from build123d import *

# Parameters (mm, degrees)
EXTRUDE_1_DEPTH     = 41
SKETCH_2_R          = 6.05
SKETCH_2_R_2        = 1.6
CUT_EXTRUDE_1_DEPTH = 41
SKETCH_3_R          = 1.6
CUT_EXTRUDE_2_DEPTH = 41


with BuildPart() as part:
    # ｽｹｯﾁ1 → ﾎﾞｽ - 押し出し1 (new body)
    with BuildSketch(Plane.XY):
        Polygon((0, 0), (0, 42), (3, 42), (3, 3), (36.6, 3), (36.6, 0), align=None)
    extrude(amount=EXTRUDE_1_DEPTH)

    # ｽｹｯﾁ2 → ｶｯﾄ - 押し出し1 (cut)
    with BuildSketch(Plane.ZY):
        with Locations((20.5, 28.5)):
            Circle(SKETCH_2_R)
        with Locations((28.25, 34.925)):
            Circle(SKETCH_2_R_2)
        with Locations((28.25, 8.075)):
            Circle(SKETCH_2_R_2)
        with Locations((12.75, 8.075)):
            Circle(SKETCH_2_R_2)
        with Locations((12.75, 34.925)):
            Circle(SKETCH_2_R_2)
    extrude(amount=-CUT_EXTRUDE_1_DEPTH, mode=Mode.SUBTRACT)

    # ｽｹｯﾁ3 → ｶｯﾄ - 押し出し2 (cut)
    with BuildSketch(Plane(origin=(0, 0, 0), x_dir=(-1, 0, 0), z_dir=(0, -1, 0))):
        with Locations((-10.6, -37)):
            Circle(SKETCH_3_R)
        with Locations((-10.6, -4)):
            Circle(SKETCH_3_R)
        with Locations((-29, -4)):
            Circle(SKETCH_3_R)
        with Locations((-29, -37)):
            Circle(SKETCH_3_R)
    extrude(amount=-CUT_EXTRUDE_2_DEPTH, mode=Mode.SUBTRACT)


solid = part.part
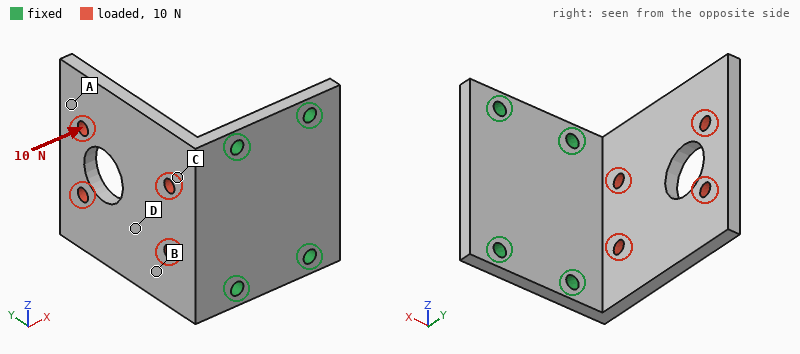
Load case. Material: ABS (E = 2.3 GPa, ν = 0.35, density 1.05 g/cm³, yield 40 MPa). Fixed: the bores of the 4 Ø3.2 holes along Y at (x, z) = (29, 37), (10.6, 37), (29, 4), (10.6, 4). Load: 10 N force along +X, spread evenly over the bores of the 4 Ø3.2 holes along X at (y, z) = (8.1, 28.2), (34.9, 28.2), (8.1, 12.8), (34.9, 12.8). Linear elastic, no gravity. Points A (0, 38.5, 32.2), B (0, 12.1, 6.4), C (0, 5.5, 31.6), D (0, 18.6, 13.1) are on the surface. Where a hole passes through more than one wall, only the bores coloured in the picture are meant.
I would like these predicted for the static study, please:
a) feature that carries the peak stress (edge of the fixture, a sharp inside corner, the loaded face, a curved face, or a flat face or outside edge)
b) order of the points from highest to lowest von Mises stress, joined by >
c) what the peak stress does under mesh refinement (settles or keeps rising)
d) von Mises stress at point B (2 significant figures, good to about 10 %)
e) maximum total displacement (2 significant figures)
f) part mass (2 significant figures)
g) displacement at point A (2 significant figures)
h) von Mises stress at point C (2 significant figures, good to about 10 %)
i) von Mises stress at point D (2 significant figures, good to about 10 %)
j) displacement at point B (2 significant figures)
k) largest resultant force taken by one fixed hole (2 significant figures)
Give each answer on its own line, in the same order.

edge of the fixture
C > B > D > A
keeps rising
1.9 MPa
0.74 mm
9.2 g
0.65 mm
2.5 MPa
1.2 MPa
0.14 mm
3.6 N
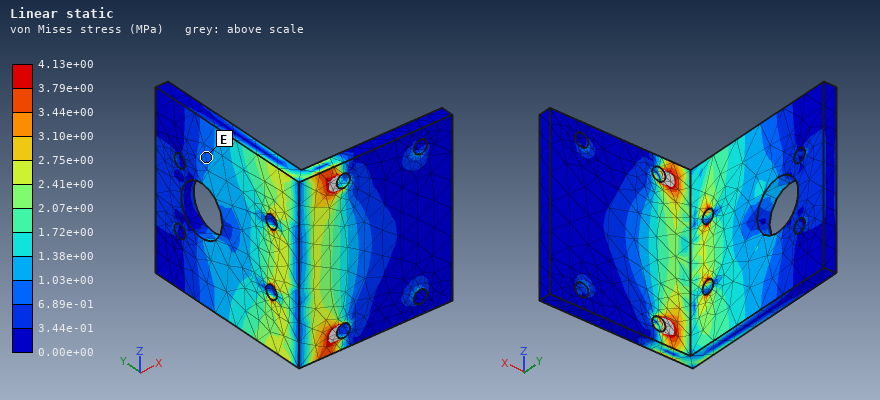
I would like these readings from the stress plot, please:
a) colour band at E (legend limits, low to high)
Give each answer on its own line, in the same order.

6.89e-01 to 1.03e+00 MPa
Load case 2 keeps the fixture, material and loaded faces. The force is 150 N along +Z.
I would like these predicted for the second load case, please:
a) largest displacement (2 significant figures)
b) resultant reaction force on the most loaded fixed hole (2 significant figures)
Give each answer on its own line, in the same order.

0.77 mm
120 N
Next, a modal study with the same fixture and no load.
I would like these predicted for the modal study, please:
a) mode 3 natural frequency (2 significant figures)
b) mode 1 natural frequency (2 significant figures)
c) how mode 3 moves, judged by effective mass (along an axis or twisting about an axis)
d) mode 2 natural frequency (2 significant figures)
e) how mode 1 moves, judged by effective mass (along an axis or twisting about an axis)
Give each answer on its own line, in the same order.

1400 Hz
340 Hz
along Z
860 Hz
along X
